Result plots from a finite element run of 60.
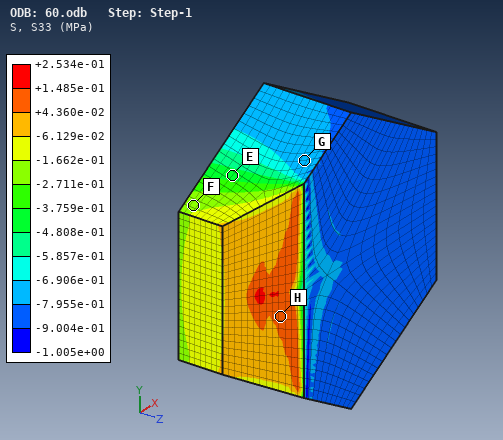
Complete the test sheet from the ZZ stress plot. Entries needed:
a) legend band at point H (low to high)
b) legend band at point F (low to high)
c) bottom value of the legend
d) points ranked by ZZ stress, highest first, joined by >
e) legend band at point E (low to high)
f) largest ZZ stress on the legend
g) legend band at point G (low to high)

+4.360e-02 to +1.485e-01 MPa
-2.711e-01 to -1.662e-01 MPa
-1.005e+00 MPa
H > F > E > G
-4.808e-01 to -3.759e-01 MPa
+2.534e-01 MPa
-7.955e-01 to -6.906e-01 MPa
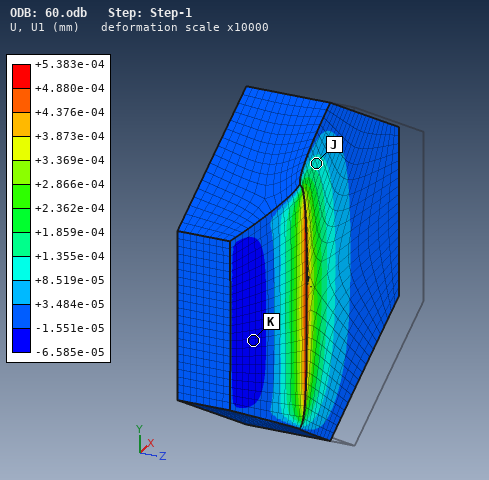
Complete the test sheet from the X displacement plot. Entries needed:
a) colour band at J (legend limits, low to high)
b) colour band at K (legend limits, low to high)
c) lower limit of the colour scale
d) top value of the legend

+8.519e-05 to +1.355e-04 mm
-6.585e-05 to -1.551e-05 mm
-6.585e-05 mm
+5.383e-04 mm
